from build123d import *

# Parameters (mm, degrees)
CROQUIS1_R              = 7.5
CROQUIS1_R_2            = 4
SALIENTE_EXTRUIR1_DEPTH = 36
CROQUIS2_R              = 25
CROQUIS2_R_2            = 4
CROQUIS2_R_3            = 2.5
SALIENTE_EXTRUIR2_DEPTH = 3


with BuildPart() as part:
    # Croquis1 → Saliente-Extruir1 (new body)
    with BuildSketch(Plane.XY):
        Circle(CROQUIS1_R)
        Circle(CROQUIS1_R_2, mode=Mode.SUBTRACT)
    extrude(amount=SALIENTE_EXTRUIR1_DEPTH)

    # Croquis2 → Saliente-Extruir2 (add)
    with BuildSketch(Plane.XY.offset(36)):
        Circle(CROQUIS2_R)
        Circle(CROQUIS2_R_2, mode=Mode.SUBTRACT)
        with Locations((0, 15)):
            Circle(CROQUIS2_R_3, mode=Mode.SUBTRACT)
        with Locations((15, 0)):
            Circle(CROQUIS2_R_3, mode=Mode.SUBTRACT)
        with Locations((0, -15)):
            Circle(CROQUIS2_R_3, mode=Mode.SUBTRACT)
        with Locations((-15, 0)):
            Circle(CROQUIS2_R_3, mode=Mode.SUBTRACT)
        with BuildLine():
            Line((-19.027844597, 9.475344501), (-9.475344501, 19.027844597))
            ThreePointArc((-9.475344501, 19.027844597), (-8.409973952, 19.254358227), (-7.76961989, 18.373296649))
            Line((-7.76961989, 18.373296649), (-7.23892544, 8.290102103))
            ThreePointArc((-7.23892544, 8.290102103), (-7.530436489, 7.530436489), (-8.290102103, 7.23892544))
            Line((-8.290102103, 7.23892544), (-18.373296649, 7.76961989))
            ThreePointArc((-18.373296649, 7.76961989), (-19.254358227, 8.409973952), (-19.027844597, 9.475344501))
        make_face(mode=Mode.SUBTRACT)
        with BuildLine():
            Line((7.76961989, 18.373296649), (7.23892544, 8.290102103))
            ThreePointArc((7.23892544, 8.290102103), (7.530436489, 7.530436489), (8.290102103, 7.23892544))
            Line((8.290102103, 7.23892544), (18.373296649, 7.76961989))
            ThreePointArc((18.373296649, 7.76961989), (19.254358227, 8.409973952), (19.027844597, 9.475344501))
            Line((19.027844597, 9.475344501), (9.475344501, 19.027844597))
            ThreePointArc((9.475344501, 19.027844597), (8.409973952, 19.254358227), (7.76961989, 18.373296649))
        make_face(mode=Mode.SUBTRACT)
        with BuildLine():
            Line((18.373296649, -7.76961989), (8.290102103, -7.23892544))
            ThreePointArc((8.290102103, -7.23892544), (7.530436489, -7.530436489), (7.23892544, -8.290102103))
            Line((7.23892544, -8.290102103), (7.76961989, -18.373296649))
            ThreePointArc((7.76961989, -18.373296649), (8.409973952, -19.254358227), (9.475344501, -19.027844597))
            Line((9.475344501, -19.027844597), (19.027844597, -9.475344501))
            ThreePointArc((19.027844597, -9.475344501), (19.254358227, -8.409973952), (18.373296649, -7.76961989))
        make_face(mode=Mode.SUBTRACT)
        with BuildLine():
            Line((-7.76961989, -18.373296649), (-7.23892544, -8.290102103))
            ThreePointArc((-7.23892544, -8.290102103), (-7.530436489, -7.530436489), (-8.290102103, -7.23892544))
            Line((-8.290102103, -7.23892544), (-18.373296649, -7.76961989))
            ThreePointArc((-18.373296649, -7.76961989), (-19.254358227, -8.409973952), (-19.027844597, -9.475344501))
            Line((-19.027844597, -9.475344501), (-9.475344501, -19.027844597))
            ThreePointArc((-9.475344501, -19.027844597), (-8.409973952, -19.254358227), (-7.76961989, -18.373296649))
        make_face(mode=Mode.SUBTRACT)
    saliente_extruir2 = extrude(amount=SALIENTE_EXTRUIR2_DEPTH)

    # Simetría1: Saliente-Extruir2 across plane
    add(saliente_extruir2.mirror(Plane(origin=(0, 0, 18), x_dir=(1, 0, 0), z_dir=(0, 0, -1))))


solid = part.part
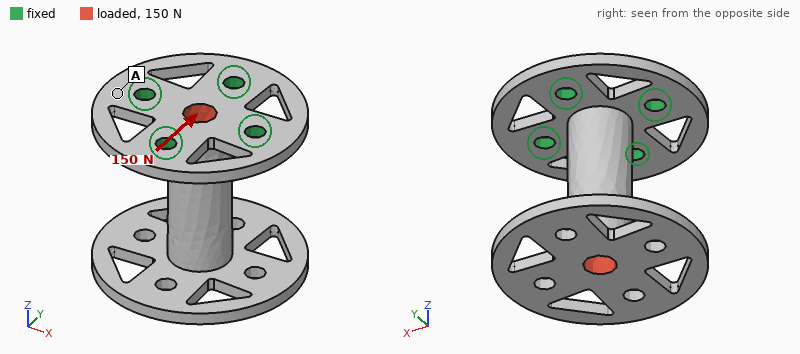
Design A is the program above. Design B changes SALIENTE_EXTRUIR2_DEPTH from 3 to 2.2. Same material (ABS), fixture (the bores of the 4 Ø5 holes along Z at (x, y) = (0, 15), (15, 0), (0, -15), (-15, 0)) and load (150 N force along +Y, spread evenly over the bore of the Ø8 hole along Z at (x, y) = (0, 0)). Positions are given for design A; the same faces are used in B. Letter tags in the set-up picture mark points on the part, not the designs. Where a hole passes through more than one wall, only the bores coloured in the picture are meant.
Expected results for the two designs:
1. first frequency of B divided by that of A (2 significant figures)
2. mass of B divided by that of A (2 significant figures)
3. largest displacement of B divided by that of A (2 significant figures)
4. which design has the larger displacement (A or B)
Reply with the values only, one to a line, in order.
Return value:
0.92
0.82
1.5
B
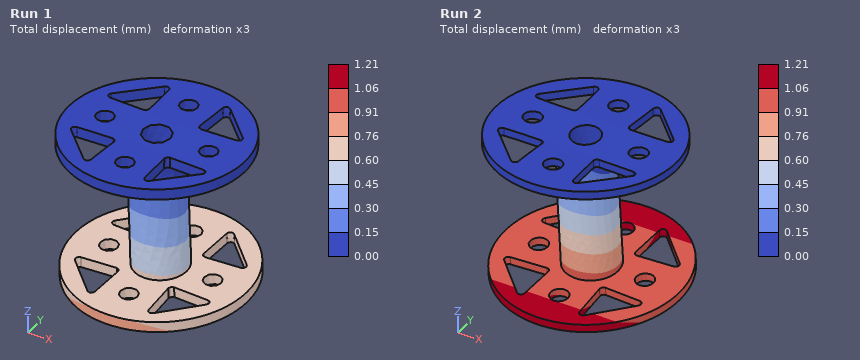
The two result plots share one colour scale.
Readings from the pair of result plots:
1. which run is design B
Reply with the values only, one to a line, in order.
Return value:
Run 2
